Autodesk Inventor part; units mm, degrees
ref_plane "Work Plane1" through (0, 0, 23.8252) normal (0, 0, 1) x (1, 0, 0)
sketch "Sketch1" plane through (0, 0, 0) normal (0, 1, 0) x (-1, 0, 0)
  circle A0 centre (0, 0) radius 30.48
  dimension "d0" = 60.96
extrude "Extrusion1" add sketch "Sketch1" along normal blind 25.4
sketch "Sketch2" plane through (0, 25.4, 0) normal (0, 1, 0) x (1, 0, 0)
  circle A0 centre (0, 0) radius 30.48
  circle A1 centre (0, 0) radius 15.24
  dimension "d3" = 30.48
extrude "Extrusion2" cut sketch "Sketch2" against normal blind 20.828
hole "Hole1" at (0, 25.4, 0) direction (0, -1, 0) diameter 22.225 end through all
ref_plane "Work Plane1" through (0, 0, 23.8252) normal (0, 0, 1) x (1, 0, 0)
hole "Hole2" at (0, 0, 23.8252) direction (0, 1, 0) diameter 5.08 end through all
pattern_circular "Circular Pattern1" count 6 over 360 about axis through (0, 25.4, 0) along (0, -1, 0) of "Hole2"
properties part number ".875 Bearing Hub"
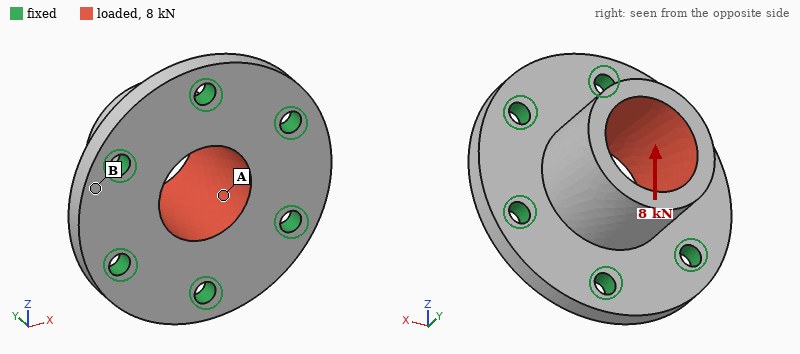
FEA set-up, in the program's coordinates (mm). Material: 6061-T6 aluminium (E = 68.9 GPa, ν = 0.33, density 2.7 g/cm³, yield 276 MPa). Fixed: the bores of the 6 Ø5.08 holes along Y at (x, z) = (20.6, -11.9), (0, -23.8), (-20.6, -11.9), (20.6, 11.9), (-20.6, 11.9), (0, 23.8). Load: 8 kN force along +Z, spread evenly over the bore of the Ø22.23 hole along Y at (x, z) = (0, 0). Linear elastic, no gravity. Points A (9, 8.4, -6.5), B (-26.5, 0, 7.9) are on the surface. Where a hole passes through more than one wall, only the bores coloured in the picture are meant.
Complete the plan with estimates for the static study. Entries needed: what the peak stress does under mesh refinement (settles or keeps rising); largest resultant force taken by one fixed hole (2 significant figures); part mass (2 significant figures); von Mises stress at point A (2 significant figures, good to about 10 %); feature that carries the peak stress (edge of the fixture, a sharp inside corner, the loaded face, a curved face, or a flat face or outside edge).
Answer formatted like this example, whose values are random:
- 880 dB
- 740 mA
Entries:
- keeps rising
- 2.4 kN
- 49 g
- 38 MPa
- edge of the fixture
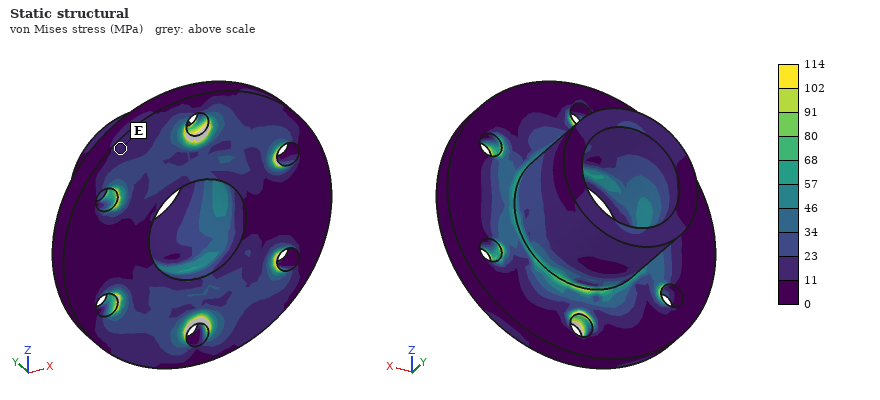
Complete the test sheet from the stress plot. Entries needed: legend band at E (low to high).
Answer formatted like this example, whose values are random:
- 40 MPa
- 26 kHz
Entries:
- 11 to 23 MPa
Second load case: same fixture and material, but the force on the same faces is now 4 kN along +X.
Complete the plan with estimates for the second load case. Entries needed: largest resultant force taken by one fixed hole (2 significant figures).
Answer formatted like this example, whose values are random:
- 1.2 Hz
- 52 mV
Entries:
- 1.0 kN
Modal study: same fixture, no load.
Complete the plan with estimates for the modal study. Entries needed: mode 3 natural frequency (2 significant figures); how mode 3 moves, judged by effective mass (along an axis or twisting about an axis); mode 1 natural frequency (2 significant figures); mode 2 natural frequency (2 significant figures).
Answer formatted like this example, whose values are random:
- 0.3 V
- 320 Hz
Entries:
- 18 kHz
- along Y
- 14 kHz
- 14 kHz
